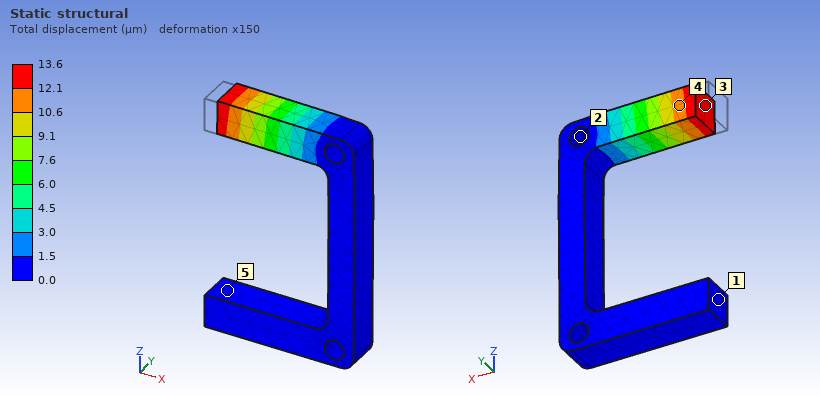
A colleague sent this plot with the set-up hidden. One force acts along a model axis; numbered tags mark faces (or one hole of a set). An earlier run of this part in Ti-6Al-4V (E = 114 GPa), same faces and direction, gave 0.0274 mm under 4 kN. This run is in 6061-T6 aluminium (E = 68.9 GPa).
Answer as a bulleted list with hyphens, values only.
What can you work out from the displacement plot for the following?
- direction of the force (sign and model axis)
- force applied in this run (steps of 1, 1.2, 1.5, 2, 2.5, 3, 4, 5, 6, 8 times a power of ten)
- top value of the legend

- +X
- 1.2 kN
- 13.6 µm
